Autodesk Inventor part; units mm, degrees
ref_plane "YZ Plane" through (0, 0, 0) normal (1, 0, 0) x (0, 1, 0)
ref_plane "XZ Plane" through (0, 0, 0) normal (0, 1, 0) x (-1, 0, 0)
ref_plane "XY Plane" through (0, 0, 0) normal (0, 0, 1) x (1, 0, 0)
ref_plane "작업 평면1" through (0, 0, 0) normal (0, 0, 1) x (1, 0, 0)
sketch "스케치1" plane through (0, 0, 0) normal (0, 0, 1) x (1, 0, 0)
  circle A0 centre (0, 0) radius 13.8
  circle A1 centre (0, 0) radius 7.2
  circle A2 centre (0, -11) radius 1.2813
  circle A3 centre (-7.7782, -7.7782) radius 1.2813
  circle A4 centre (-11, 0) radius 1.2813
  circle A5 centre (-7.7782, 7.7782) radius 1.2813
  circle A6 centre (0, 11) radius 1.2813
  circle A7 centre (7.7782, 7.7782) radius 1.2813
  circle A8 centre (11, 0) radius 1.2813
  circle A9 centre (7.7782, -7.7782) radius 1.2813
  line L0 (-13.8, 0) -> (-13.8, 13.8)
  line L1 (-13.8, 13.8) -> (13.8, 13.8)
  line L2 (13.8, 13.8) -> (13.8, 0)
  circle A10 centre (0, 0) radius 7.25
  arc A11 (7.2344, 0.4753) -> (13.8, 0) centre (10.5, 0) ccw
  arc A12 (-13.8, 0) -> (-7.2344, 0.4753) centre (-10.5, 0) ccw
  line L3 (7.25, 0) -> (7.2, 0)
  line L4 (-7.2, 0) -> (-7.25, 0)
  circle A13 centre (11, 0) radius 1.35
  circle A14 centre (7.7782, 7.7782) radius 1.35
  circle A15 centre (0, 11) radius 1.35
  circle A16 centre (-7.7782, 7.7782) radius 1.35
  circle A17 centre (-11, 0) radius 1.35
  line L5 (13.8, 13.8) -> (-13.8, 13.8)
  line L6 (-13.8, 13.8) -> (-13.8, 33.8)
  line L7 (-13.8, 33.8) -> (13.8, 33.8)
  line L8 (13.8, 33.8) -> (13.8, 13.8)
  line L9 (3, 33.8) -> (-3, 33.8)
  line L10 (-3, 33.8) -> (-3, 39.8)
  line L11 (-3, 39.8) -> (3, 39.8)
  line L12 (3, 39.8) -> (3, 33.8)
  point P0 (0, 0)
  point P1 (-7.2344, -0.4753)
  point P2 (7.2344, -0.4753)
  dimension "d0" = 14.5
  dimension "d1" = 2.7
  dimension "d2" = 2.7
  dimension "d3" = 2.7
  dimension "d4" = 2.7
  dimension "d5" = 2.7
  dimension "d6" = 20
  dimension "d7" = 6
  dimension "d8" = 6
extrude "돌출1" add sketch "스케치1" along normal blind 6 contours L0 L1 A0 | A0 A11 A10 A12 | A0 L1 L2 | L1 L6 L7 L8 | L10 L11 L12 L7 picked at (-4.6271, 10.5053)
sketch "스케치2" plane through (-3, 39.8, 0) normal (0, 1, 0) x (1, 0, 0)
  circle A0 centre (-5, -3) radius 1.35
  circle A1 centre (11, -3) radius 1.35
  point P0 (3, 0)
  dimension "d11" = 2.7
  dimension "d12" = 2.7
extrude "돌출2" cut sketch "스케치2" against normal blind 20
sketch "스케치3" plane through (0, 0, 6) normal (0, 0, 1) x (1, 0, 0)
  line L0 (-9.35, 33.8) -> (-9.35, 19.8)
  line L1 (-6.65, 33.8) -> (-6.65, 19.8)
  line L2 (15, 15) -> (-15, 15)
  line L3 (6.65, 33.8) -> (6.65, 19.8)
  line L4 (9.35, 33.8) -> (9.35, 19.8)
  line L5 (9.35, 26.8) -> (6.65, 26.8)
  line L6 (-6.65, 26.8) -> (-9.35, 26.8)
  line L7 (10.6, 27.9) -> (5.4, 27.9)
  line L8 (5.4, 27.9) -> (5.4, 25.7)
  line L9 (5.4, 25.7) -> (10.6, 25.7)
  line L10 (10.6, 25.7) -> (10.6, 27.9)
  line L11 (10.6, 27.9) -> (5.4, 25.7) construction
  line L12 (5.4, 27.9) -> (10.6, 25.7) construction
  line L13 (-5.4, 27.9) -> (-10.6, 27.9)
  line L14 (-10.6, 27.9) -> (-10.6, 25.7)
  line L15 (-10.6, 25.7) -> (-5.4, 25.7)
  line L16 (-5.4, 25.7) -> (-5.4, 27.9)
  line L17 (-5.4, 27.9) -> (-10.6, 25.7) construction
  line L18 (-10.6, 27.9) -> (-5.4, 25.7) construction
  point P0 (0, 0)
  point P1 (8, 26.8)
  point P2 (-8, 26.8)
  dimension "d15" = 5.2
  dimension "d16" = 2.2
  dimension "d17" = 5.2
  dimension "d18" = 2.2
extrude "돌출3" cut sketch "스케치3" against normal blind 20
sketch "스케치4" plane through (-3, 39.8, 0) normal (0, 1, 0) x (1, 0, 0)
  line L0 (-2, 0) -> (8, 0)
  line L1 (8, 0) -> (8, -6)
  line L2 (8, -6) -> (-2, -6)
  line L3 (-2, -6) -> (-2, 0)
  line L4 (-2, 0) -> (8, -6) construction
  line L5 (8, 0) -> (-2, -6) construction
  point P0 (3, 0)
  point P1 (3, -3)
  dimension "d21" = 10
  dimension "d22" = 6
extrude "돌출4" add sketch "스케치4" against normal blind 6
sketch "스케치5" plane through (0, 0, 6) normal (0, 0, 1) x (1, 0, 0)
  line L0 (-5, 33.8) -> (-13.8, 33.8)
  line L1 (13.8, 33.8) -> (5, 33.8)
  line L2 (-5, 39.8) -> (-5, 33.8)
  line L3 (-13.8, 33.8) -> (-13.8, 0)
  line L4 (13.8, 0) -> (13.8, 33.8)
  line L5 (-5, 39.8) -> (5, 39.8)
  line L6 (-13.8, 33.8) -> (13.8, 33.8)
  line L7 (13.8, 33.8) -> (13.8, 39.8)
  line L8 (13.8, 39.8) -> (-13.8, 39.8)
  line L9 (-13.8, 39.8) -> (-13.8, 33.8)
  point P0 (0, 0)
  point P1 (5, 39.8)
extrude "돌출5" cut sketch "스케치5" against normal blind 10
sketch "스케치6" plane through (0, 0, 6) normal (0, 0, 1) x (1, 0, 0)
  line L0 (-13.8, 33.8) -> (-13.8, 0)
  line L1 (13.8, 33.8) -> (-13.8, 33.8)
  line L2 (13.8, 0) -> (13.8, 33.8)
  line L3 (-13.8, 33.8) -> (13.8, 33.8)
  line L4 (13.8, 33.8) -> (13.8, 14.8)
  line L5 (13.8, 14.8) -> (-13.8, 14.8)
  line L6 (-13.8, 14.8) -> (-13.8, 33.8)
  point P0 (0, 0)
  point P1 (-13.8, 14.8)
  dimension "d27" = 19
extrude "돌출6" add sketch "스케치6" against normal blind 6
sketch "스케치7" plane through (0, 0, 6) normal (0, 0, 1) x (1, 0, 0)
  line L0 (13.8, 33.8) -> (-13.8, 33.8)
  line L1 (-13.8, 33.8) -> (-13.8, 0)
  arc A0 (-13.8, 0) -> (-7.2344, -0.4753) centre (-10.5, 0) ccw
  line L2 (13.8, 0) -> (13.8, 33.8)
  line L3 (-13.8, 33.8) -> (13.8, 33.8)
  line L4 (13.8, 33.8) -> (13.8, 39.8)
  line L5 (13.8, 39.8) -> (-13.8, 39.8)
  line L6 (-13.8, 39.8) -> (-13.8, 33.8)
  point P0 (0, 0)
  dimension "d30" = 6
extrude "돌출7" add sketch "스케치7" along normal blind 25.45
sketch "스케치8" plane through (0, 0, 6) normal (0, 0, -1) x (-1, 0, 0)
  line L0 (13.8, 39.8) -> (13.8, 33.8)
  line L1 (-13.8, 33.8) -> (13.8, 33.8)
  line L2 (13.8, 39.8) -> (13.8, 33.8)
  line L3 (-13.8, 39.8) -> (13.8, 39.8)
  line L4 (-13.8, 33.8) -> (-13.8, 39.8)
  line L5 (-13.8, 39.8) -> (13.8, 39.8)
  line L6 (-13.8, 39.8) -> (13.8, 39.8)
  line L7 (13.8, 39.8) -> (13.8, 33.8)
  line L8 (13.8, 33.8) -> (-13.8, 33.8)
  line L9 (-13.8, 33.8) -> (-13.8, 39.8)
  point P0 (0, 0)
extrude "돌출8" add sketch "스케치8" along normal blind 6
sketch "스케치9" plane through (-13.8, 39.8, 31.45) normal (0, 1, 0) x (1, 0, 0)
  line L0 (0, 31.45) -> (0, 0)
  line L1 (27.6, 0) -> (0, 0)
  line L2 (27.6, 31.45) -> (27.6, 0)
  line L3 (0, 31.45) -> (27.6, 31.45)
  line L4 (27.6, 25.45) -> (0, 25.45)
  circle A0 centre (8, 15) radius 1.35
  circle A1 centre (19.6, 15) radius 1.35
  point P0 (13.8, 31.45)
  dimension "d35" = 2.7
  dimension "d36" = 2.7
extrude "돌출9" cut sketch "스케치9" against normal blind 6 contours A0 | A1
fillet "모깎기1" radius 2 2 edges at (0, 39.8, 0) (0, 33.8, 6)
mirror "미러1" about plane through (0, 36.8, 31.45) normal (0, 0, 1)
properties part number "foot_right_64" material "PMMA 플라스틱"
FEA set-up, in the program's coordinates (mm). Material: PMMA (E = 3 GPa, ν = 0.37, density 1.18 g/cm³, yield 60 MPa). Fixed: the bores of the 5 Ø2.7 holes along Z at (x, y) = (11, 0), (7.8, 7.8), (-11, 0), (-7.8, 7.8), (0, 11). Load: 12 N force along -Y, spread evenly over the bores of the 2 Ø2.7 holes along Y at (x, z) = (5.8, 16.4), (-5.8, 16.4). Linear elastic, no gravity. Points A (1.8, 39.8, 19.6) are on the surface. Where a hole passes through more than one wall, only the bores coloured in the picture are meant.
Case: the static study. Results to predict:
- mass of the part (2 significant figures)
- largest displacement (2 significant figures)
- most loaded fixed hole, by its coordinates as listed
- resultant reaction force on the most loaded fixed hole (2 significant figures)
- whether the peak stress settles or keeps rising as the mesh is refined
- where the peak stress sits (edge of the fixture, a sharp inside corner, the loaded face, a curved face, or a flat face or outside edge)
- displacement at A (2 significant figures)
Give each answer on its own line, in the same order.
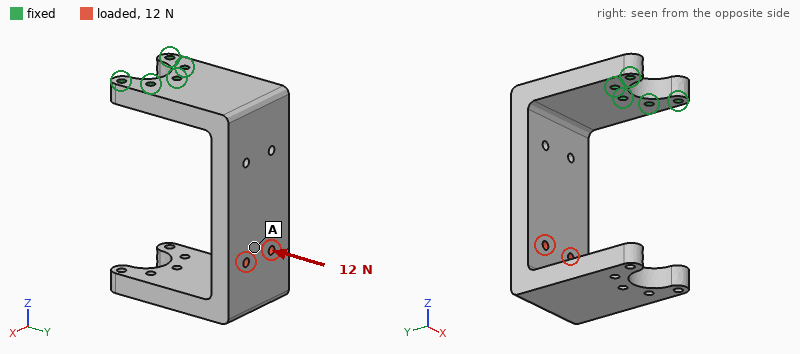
24 g
0.95 mm
(0, 11)
24 N
keeps rising
edge of the fixture
0.54 mm
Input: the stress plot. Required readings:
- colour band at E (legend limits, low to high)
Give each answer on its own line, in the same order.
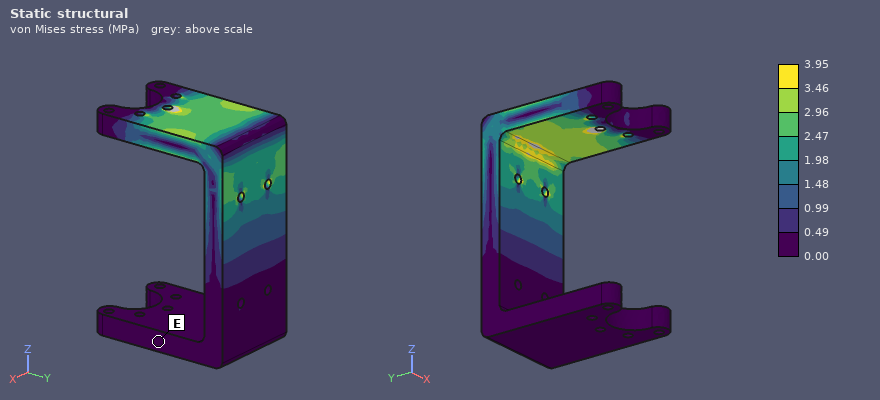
0.00 to 0.49 MPa
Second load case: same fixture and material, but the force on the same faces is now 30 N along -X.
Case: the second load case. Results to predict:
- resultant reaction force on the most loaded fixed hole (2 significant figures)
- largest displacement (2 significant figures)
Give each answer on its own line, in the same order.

62 N
0.92 mm
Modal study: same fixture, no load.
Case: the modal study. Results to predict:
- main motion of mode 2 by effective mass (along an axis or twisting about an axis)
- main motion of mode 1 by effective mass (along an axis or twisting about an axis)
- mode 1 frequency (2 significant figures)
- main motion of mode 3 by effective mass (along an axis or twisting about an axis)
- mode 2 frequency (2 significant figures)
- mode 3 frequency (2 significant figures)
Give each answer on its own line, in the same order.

along X
along Y
160 Hz
along Z
240 Hz
530 Hz
